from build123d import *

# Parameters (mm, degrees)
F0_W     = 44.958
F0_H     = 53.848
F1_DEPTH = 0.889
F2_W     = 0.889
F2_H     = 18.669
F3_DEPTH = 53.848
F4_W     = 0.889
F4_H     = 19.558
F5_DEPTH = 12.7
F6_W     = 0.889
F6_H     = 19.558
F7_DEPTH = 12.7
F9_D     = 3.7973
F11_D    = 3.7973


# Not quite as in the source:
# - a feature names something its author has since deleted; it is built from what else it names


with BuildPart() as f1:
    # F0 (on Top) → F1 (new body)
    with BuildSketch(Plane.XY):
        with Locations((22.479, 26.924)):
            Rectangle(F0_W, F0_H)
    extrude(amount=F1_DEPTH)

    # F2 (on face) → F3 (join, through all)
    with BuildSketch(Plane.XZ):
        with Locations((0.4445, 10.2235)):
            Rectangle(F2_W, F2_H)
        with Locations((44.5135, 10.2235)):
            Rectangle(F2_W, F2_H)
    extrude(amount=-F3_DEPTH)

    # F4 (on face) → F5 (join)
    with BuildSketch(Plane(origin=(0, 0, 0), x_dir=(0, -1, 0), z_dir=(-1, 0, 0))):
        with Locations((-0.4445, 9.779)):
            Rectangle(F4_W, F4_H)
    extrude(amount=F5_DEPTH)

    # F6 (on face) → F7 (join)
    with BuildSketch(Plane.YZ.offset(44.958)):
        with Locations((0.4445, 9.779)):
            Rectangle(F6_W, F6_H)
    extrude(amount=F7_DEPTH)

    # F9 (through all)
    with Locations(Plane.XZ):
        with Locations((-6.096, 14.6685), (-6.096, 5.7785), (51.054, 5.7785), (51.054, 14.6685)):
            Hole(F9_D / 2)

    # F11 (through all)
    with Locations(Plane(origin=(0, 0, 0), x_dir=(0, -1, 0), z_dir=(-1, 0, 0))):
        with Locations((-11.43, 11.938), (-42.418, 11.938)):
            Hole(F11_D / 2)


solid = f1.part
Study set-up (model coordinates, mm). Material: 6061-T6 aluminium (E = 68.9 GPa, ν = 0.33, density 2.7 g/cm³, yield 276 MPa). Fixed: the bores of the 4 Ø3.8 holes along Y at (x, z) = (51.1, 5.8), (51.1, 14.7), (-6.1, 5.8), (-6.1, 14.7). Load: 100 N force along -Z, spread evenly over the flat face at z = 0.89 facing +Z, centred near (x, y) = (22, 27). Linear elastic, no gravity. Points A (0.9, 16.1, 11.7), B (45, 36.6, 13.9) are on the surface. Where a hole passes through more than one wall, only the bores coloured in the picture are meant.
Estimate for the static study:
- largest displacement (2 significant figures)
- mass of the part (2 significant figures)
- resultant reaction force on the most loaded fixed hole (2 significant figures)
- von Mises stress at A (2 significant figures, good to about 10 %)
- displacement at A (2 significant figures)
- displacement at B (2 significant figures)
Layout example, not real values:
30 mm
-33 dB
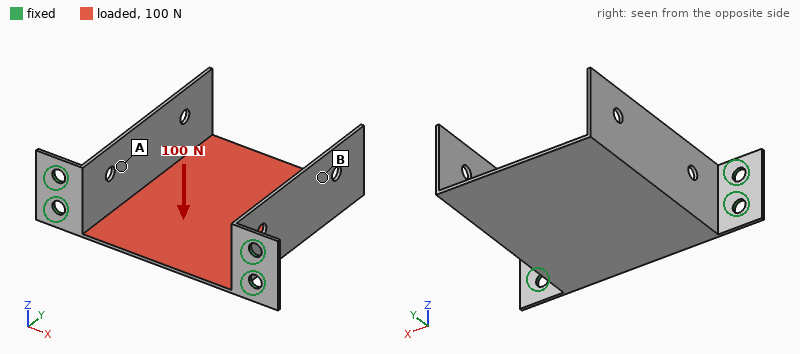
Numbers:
0.95 mm
12 g
130 N
36 MPa
0.18 mm
0.44 mm
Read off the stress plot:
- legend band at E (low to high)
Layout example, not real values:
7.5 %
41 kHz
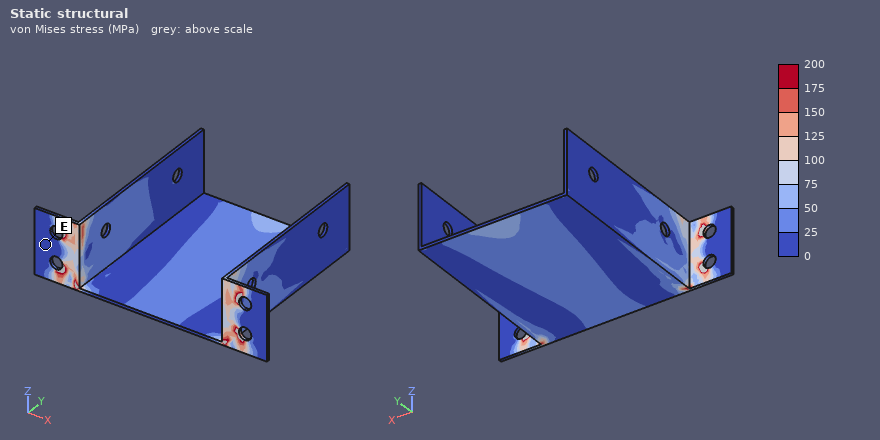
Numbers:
0 to 25 MPa
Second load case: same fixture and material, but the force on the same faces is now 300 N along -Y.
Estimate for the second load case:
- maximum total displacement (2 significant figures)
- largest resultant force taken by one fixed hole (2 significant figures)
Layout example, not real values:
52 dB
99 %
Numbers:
0.57 mm
220 N
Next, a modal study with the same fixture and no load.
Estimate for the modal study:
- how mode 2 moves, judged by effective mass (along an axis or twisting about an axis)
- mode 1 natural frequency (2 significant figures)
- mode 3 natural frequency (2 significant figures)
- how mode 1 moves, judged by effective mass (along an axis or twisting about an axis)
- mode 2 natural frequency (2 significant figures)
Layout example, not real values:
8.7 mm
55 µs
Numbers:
along X
710 Hz
1100 Hz
along Z
820 Hz
